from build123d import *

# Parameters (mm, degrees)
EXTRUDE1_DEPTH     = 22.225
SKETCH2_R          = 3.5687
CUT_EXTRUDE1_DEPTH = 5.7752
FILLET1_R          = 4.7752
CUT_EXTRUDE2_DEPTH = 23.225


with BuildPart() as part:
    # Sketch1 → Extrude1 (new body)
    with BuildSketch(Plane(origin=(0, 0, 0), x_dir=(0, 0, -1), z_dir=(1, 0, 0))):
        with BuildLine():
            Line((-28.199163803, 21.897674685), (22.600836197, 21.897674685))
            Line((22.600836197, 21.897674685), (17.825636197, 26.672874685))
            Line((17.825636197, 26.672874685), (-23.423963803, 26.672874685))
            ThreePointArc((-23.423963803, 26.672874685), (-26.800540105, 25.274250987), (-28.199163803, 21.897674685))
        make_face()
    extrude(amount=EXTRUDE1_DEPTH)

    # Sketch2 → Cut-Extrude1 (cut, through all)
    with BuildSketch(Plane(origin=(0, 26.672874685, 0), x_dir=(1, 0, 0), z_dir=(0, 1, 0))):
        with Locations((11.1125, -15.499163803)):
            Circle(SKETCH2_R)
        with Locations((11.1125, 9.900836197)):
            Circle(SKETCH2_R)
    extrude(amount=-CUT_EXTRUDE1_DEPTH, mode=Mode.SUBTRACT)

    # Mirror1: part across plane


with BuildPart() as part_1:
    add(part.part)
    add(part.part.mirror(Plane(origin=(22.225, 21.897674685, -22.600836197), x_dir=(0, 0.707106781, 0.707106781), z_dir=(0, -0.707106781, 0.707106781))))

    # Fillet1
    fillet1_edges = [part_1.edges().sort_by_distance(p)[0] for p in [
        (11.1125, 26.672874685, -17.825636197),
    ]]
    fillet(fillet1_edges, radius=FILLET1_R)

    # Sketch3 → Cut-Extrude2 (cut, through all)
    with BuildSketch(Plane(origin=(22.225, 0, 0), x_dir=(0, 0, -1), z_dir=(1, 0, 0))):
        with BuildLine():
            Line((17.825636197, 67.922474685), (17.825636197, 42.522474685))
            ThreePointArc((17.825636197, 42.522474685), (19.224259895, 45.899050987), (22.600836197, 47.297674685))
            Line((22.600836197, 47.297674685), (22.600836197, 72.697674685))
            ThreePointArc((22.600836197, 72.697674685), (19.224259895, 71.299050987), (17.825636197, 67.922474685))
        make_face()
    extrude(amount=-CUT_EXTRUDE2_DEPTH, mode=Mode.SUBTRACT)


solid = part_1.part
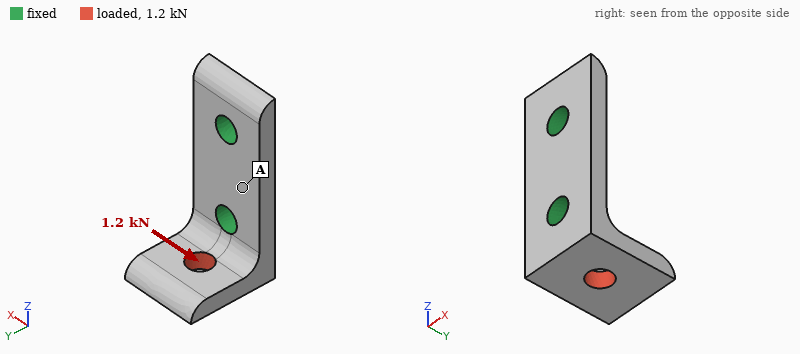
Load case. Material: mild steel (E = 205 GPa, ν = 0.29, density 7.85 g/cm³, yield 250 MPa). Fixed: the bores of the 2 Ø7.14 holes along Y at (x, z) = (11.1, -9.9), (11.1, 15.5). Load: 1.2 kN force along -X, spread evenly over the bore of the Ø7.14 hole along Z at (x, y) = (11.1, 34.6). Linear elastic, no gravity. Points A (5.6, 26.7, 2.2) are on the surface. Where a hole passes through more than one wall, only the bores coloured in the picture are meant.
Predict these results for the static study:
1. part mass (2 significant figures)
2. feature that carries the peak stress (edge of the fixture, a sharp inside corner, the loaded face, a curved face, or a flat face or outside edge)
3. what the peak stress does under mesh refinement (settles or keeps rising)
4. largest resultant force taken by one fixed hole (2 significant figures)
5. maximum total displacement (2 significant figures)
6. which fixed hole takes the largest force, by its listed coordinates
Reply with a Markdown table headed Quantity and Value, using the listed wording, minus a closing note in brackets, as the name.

| Quantity | Value |
|---|---|
| part mass | 54 g |
| feature that carries the peak stress | edge of the fixture |
| what the peak stress does under mesh refinement | keeps rising |
| largest resultant force taken by one fixed hole | 1.4 kN |
| maximum total displacement | 27 µm |
| which fixed hole takes the largest force, by its listed coordinates | (11.1, -9.9) |
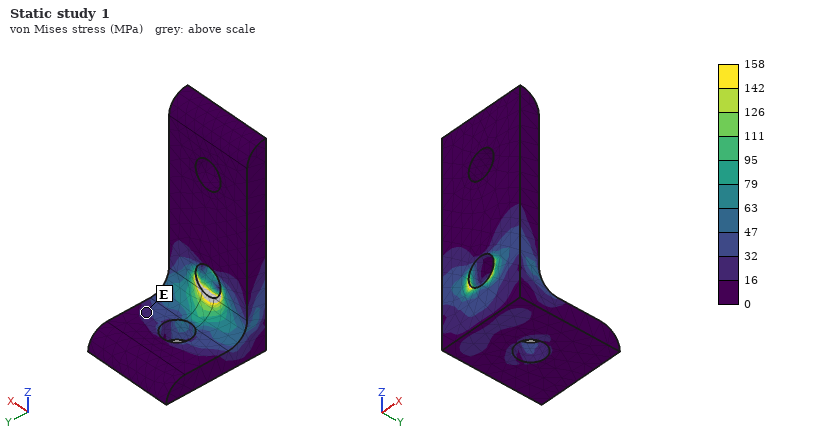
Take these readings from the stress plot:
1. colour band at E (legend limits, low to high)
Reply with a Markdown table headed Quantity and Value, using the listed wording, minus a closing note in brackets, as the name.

| Quantity | Value |
|---|---|
| colour band at E | 16 to 32 MPa |
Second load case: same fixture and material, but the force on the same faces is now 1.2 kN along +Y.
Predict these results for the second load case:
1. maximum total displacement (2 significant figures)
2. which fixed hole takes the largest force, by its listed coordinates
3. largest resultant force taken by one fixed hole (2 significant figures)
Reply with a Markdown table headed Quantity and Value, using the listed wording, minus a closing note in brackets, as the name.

| Quantity | Value |
|---|---|
| maximum total displacement | 25 µm |
| which fixed hole takes the largest force, by its listed coordinates | (11.1, -9.9) |
| largest resultant force taken by one fixed hole | 1.2 kN |
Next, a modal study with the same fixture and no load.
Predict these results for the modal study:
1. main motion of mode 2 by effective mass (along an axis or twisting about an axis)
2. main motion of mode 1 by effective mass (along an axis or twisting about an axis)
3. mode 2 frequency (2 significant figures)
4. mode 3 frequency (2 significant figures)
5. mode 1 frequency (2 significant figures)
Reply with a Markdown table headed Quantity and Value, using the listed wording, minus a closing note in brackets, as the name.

| Quantity | Value |
|---|---|
| main motion of mode 2 by effective mass | along X |
| main motion of mode 1 by effective mass | along Z |
| mode 2 frequency | 8800 Hz |
| mode 3 frequency | 16 kHz |
| mode 1 frequency | 6100 Hz |
